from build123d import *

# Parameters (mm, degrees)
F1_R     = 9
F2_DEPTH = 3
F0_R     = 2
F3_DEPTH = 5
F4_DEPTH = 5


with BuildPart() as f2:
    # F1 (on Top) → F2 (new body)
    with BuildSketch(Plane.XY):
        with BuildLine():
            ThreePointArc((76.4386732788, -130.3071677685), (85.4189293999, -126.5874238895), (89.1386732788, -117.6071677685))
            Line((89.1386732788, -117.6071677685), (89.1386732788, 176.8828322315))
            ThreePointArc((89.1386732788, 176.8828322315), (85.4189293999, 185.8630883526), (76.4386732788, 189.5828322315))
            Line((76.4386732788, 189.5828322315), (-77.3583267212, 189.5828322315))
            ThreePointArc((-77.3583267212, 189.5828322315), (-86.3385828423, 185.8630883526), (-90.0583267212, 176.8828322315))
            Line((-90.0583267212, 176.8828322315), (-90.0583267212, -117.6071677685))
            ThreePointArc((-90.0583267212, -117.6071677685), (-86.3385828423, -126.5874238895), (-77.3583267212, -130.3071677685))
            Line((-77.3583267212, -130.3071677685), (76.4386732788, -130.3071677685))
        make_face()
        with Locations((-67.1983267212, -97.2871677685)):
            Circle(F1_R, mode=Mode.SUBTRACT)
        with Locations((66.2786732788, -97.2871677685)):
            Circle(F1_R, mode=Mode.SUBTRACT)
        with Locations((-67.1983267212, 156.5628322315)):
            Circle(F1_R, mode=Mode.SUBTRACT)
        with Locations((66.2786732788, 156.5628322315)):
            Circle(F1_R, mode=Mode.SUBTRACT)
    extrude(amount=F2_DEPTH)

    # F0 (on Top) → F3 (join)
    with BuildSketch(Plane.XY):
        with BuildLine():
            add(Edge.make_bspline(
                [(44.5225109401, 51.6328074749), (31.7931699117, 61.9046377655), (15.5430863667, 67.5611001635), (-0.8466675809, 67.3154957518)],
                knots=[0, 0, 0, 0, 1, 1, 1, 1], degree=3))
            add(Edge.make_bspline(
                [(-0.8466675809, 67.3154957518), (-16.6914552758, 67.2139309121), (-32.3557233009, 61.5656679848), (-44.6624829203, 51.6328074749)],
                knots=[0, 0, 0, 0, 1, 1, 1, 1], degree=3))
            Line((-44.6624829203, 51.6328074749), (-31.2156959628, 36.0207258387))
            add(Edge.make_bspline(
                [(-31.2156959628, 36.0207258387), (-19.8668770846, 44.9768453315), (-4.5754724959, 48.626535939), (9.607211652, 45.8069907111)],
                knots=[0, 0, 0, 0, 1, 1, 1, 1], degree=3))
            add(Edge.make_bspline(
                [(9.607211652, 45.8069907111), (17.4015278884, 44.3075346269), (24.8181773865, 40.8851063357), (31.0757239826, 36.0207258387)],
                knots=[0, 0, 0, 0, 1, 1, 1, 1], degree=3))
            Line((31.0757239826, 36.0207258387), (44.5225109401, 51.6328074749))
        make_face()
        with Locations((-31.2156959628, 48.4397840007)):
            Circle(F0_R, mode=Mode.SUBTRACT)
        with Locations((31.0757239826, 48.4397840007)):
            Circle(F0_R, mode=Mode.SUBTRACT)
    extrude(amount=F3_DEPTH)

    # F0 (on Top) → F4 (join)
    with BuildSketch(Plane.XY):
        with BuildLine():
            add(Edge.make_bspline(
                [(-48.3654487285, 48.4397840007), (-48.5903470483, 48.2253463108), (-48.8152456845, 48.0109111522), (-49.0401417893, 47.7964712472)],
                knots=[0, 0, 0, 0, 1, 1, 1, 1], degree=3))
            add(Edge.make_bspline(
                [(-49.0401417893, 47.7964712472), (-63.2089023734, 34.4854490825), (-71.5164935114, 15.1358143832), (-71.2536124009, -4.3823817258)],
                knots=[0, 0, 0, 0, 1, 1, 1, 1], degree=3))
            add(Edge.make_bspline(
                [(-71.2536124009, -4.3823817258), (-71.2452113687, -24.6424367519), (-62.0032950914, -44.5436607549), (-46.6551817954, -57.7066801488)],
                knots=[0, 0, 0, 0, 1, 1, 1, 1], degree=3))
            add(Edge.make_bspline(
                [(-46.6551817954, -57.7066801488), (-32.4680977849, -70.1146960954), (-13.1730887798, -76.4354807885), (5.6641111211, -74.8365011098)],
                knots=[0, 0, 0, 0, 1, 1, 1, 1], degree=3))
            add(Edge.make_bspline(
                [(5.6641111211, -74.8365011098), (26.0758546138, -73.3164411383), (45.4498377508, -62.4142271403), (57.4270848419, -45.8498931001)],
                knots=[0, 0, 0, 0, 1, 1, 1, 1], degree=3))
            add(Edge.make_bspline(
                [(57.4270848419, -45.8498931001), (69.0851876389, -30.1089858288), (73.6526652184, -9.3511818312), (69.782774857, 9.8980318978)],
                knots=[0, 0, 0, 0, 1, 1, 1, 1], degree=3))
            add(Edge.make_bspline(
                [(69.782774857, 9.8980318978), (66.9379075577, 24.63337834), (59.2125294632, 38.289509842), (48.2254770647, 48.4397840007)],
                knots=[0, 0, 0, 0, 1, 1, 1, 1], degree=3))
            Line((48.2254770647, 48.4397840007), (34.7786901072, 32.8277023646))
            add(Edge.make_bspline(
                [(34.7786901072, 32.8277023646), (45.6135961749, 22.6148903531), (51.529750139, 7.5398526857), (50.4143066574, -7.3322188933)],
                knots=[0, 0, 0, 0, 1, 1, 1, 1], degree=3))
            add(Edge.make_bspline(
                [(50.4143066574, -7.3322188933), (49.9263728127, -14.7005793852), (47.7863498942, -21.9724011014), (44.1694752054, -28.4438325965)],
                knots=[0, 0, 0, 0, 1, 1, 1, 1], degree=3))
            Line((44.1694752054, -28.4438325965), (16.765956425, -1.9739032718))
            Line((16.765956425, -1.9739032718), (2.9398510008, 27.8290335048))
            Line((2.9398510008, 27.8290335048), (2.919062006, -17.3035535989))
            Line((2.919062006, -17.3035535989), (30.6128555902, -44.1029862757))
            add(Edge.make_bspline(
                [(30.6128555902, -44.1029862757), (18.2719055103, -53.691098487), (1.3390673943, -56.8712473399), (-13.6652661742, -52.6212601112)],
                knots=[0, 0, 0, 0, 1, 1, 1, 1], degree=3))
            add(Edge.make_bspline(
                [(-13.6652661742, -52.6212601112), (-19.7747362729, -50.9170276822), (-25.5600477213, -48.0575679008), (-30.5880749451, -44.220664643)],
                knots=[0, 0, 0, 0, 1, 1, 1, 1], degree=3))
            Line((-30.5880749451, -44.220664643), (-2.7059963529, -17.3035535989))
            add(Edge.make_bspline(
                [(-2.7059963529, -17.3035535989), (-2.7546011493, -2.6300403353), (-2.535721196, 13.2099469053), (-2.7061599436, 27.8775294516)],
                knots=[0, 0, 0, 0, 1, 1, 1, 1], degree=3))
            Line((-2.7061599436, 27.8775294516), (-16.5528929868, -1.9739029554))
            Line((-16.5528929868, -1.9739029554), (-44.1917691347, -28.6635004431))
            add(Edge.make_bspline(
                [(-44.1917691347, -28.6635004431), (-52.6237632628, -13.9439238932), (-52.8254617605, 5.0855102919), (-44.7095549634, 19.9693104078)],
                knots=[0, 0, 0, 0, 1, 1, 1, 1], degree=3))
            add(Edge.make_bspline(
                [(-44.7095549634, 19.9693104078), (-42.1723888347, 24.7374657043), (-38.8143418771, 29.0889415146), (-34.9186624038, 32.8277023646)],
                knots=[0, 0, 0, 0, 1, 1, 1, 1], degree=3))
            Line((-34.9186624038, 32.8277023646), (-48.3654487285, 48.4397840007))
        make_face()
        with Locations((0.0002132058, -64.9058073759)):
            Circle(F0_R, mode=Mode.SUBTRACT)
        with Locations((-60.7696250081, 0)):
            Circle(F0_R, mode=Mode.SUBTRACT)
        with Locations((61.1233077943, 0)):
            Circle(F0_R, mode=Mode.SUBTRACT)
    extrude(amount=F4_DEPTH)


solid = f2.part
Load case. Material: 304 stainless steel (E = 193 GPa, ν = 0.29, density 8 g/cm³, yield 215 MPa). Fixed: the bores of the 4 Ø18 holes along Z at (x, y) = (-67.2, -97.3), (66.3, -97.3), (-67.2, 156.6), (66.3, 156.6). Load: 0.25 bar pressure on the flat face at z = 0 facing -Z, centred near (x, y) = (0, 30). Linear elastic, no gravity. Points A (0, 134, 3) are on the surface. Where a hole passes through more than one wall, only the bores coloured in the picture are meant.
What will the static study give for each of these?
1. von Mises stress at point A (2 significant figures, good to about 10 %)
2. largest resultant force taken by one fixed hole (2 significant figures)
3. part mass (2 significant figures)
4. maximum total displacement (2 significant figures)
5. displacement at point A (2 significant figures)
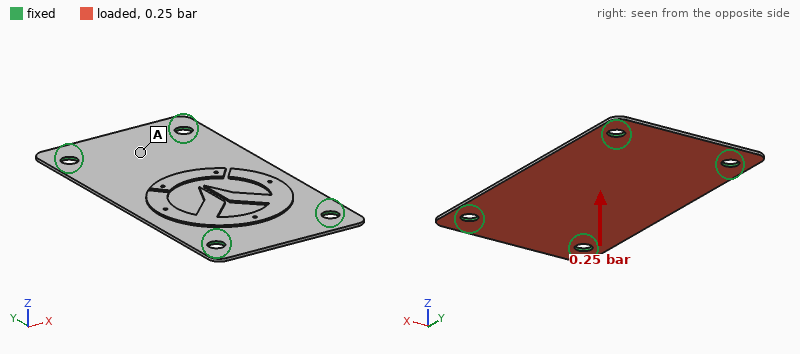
26 MPa
550 N
1.5 kg
0.46 mm
0.14 mm
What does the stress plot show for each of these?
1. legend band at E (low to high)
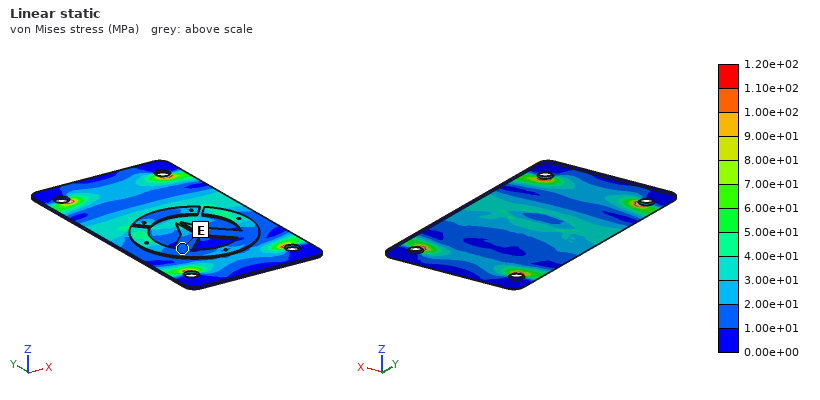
1.00e+01 to 2.00e+01 MPa
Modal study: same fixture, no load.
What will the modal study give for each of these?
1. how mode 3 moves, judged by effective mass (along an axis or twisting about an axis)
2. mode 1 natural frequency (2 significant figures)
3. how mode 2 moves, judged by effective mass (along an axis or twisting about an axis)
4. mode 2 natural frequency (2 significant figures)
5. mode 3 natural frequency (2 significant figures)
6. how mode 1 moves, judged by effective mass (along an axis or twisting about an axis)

twisting about X
250 Hz
twisting about Y
390 Hz
700 Hz
along Z
